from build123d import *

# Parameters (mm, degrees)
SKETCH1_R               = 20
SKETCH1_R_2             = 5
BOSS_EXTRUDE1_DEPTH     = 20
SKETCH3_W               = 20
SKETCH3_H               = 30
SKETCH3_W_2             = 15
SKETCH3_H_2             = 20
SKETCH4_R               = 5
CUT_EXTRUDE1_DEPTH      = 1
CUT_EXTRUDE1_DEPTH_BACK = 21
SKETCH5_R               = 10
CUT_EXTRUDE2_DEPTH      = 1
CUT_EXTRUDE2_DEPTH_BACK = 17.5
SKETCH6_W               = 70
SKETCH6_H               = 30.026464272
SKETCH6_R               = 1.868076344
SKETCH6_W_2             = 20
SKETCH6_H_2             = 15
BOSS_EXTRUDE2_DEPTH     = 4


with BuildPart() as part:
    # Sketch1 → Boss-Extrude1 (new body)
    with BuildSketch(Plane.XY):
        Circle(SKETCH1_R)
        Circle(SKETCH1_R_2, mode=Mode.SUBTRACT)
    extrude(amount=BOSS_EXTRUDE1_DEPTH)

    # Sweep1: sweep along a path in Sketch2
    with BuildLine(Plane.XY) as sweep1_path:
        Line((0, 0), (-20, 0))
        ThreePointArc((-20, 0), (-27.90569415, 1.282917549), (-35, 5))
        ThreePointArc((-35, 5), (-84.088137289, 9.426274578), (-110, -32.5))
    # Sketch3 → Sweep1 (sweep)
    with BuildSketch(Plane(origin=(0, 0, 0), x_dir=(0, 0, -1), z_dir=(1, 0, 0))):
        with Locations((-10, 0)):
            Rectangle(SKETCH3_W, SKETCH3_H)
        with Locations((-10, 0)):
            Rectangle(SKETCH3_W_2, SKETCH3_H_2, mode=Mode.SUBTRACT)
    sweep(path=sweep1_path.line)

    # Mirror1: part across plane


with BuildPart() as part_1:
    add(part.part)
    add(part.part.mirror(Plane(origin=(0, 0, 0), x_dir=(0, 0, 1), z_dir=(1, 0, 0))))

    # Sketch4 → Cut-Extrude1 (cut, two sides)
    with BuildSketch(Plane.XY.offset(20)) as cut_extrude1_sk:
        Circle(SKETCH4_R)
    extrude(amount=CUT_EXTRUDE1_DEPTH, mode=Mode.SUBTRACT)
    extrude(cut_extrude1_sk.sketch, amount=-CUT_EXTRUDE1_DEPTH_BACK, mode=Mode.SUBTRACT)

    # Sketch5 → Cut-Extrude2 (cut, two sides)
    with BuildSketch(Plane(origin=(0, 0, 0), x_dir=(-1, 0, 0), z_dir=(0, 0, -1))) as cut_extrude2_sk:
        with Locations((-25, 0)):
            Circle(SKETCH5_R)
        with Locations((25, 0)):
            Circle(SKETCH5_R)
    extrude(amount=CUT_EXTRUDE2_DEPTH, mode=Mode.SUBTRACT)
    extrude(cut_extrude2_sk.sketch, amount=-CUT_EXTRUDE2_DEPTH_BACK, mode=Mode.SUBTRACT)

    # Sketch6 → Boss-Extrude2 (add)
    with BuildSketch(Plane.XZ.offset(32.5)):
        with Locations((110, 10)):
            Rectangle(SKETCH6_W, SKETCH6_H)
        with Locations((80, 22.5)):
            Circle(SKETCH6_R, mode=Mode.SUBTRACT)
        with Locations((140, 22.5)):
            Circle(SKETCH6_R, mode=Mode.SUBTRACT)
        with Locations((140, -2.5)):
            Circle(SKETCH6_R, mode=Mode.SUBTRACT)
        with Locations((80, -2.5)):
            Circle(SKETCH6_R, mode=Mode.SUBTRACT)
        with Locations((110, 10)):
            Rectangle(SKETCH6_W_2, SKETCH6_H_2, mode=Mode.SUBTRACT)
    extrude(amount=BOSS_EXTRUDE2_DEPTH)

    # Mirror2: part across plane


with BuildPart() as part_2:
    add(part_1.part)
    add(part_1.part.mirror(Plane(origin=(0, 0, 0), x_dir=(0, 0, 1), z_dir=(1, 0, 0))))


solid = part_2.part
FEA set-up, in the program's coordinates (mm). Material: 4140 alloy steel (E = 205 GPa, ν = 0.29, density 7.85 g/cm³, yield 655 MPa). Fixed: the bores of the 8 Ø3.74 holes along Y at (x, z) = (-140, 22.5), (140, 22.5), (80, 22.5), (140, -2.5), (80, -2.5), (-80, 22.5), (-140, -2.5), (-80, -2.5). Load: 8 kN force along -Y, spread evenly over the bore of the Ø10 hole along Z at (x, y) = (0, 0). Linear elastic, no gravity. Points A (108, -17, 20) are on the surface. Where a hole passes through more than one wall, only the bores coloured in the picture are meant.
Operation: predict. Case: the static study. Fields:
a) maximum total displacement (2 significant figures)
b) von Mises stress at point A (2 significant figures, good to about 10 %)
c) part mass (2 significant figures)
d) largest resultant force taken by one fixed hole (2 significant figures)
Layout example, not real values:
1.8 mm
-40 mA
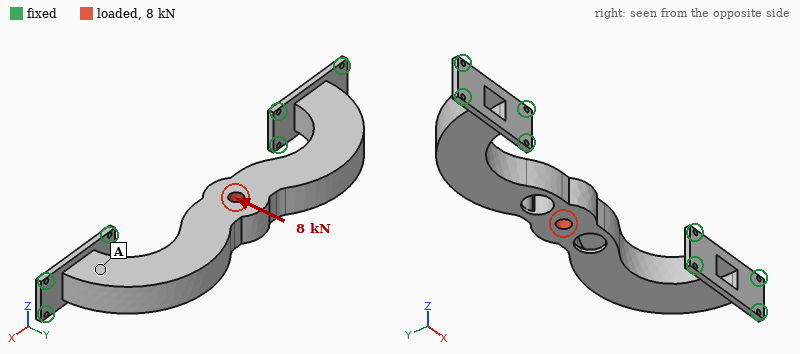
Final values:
0.18 mm
49 MPa
850 g
1.7 kN
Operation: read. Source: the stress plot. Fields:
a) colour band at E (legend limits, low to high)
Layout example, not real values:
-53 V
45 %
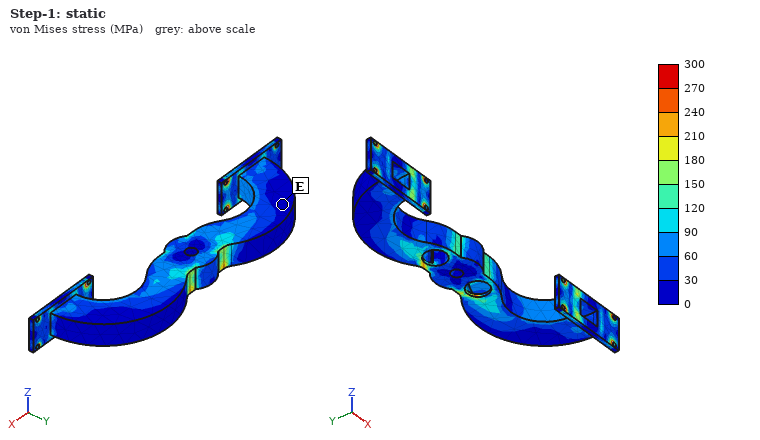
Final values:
0 to 30 MPa
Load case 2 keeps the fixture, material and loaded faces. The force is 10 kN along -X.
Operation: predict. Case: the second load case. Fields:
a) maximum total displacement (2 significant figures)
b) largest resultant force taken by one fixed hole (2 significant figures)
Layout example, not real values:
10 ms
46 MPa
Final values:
87 µm
1.7 kN
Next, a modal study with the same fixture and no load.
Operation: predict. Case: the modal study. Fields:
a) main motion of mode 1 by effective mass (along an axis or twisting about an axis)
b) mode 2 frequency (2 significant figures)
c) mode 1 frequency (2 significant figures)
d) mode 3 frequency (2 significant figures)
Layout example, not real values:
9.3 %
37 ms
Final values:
along Z
1800 Hz
690 Hz
1800 Hz
